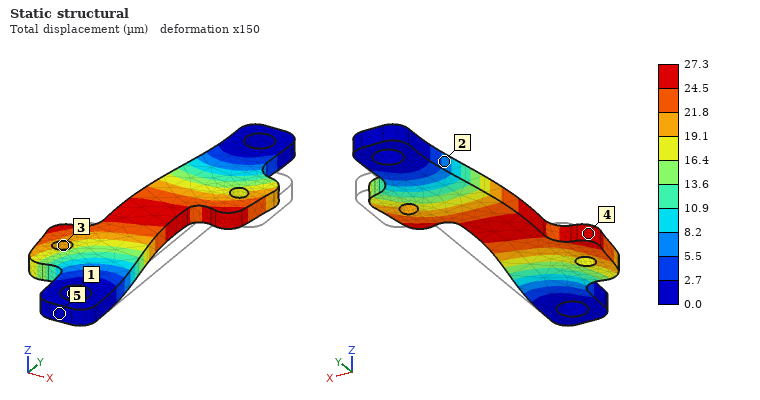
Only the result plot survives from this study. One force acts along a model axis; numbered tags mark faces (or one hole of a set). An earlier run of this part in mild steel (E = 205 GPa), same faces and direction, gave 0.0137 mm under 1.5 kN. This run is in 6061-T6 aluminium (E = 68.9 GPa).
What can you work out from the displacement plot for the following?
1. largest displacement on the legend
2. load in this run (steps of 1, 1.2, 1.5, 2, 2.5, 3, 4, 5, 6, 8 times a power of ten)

27.3 µm
1 kN
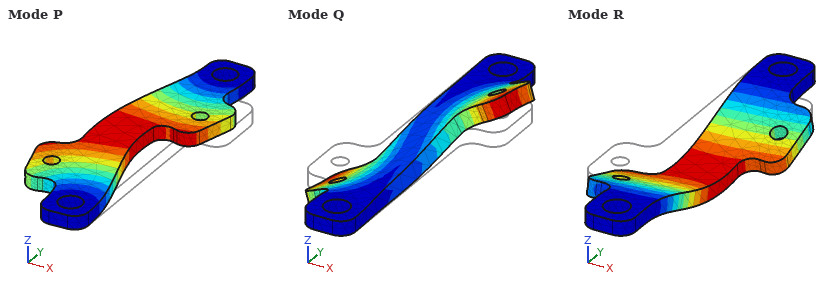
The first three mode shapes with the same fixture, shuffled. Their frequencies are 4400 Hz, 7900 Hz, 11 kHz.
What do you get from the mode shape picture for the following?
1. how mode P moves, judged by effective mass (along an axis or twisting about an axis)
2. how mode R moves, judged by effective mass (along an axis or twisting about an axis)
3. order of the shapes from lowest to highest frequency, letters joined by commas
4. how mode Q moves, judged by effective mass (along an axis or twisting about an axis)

along X
along Z
R, Q, P
twisting about Y
